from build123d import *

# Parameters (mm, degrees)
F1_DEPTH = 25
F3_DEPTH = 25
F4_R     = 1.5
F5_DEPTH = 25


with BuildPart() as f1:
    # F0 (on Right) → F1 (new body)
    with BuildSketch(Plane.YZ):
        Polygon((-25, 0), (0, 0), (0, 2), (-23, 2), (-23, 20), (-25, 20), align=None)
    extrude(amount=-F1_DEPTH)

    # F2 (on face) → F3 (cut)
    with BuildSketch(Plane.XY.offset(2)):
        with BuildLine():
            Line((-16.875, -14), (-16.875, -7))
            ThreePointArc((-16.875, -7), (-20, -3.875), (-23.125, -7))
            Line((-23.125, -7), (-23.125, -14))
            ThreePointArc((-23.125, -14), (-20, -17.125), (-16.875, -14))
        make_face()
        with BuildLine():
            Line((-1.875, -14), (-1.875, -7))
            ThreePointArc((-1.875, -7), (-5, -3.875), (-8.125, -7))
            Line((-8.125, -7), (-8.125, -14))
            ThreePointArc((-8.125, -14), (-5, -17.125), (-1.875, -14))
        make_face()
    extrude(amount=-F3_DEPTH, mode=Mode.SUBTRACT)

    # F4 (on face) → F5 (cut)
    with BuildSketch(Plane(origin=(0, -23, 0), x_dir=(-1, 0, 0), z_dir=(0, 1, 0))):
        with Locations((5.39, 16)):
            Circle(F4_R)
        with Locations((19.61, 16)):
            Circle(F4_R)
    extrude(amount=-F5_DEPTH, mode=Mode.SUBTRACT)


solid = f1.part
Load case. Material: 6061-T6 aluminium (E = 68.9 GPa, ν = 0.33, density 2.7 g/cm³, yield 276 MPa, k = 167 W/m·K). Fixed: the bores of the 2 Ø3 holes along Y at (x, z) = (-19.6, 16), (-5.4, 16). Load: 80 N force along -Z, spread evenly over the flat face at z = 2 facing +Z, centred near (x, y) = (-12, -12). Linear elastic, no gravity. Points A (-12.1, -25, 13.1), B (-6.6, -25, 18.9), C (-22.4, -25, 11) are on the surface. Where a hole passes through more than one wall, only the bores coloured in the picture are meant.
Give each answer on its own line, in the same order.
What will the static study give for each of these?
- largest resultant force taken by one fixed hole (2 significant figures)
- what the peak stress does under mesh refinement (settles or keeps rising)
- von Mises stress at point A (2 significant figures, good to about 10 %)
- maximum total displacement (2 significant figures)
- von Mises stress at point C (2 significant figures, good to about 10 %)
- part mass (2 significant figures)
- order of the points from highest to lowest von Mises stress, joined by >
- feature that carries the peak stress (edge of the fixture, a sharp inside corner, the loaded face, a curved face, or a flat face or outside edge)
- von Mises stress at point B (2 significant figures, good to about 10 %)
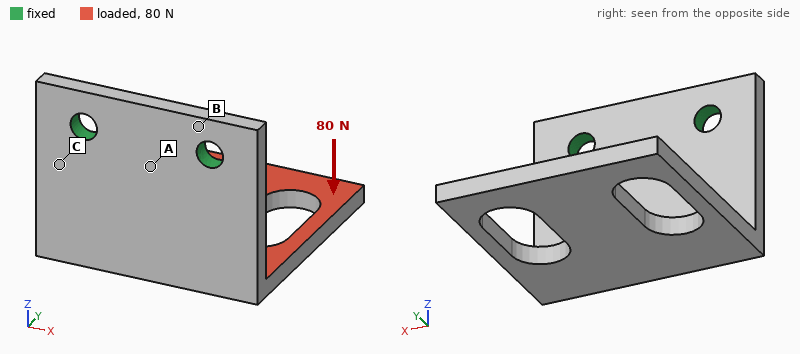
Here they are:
41 N
keeps rising
40 MPa
0.43 mm
56 MPa
4.9 g
C > A > B
edge of the fixture
12 MPa
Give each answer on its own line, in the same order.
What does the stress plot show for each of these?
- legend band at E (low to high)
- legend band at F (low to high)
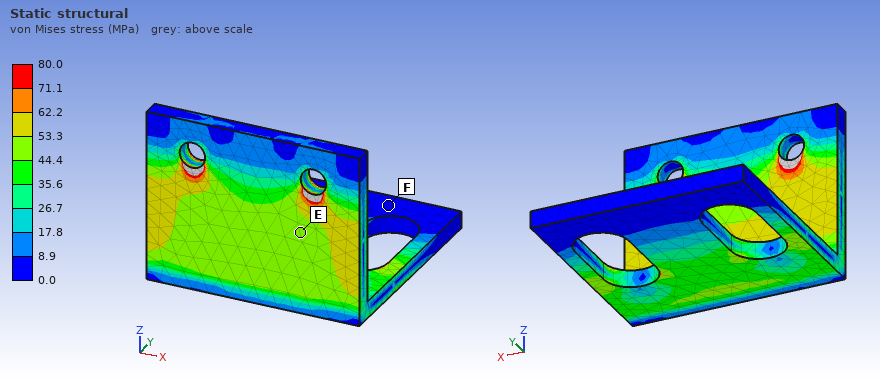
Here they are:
44.4 to 53.3 MPa
0.0 to 8.9 MPa
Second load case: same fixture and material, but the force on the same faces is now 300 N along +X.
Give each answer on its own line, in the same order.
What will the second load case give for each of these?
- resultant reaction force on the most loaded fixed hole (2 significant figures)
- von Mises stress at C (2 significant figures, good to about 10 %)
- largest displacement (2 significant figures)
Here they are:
360 N
120 MPa
0.45 mm
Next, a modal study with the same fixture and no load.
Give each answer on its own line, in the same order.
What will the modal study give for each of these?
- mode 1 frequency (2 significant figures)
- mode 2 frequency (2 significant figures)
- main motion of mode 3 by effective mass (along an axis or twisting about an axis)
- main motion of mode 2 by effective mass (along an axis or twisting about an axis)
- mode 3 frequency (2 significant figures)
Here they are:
1600 Hz
3100 Hz
along Y
along X
4600 Hz
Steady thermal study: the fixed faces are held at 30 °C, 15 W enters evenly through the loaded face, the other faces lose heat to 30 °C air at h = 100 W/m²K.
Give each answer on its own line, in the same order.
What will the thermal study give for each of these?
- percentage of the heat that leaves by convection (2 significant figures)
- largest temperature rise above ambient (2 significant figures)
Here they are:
24 %
46 K
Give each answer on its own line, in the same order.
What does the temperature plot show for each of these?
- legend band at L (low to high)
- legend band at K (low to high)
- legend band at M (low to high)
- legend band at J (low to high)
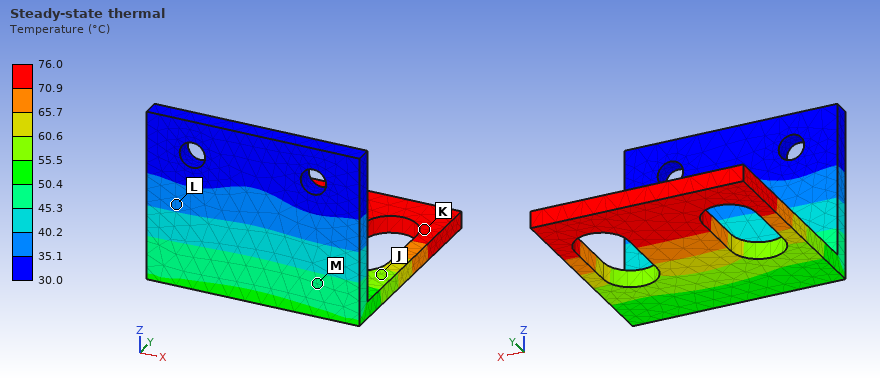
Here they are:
35.1 to 40.2 °C
70.9 to 76.0 °C
45.3 to 50.4 °C
55.5 to 60.6 °C
